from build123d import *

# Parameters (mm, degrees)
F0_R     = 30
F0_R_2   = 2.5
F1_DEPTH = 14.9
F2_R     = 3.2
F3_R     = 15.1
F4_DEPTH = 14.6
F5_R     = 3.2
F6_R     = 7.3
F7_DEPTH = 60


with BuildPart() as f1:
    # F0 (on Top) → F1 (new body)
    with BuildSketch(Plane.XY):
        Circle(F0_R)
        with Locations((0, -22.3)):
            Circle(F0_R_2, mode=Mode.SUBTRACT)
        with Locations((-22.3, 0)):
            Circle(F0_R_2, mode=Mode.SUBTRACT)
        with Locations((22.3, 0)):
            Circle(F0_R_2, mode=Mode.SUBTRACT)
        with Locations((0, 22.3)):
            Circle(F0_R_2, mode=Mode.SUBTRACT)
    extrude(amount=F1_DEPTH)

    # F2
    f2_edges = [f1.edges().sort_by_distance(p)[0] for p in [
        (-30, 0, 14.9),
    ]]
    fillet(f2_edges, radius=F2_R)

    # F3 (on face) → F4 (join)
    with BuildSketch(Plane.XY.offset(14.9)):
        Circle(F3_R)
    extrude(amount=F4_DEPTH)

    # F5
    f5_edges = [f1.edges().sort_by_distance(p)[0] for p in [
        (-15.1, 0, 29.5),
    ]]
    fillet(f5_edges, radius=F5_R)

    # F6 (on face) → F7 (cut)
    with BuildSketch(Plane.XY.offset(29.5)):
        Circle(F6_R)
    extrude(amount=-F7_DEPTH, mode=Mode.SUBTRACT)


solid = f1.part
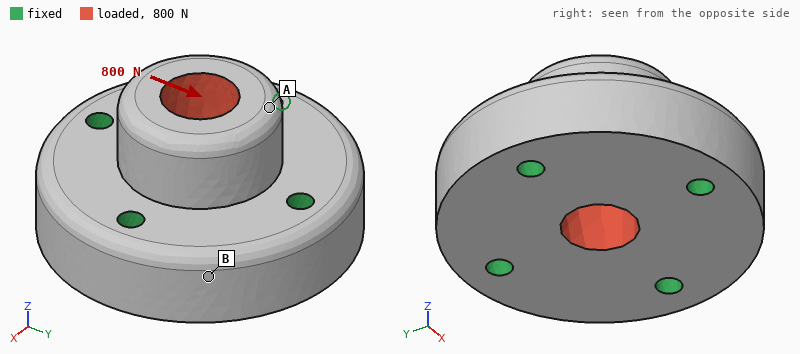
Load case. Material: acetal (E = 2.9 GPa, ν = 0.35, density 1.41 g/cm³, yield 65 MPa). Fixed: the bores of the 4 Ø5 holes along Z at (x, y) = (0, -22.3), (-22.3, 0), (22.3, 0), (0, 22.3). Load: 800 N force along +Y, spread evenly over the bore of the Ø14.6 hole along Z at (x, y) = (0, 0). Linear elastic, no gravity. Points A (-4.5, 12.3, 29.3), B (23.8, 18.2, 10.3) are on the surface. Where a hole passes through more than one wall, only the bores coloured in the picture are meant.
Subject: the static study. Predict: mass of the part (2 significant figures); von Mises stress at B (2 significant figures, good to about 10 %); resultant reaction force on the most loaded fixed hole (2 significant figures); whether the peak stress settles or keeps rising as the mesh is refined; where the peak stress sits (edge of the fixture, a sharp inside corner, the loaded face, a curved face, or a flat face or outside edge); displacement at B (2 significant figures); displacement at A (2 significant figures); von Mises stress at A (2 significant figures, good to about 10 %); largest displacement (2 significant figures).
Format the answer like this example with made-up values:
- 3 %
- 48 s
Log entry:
- 65 g
- 0.34 MPa
- 280 N
- keeps rising
- a sharp inside corner
- 3.5 µm
- 21 µm
- 0.91 MPa
- 22 µm
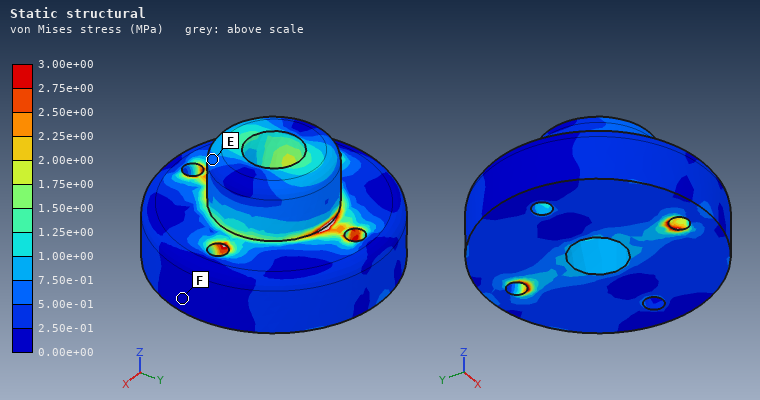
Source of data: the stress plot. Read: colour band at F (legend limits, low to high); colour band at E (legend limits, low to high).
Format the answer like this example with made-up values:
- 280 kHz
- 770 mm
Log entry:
- 0.00e+00 to 2.50e-01 MPa
- 5.00e-01 to 7.50e-01 MPa
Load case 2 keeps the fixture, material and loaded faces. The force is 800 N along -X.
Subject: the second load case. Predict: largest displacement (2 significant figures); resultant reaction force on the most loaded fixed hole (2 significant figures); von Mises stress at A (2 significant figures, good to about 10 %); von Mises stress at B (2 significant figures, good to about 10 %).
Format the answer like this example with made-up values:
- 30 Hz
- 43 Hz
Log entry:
- 22 µm
- 280 N
- 0.37 MPa
- 0.39 MPa
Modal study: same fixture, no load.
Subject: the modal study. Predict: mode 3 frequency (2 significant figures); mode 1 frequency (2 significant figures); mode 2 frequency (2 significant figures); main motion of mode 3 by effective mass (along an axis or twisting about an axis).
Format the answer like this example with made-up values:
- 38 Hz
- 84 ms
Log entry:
- 8200 Hz
- 7300 Hz
- 7300 Hz
- along Z
